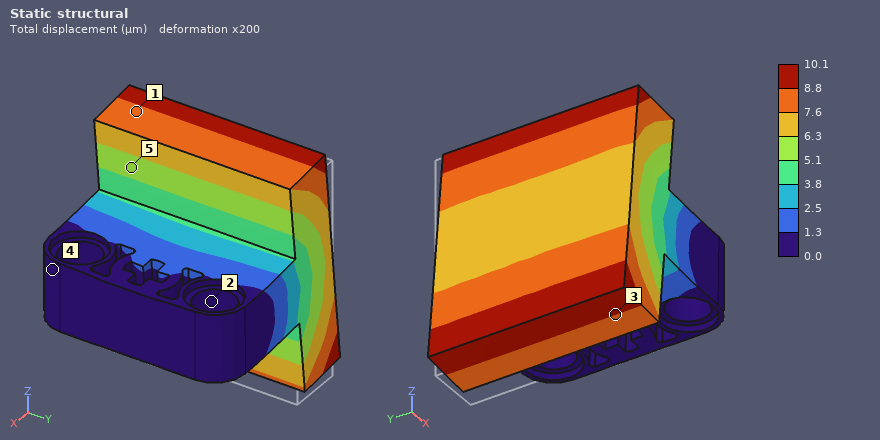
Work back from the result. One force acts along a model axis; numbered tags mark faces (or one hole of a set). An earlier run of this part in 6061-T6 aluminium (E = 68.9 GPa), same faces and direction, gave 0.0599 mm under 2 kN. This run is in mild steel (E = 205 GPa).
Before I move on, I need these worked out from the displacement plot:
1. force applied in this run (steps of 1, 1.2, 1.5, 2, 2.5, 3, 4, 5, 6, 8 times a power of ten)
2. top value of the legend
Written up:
1 kN
10.1 µm
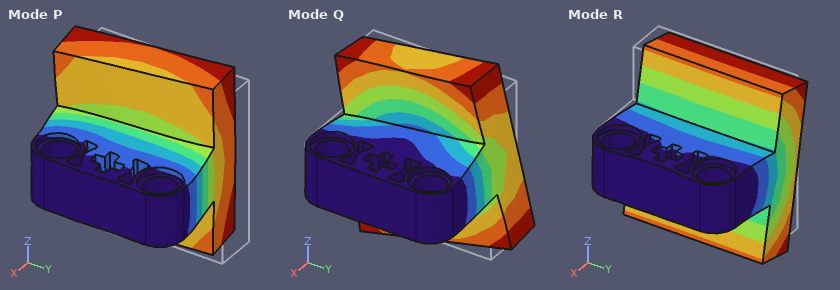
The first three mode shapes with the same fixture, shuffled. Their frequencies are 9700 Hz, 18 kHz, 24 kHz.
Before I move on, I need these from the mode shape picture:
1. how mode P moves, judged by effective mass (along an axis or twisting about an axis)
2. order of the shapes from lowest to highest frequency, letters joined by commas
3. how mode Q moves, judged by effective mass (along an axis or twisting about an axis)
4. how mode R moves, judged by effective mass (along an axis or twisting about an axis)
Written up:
along Y
R, Q, P
twisting about X
along Z
